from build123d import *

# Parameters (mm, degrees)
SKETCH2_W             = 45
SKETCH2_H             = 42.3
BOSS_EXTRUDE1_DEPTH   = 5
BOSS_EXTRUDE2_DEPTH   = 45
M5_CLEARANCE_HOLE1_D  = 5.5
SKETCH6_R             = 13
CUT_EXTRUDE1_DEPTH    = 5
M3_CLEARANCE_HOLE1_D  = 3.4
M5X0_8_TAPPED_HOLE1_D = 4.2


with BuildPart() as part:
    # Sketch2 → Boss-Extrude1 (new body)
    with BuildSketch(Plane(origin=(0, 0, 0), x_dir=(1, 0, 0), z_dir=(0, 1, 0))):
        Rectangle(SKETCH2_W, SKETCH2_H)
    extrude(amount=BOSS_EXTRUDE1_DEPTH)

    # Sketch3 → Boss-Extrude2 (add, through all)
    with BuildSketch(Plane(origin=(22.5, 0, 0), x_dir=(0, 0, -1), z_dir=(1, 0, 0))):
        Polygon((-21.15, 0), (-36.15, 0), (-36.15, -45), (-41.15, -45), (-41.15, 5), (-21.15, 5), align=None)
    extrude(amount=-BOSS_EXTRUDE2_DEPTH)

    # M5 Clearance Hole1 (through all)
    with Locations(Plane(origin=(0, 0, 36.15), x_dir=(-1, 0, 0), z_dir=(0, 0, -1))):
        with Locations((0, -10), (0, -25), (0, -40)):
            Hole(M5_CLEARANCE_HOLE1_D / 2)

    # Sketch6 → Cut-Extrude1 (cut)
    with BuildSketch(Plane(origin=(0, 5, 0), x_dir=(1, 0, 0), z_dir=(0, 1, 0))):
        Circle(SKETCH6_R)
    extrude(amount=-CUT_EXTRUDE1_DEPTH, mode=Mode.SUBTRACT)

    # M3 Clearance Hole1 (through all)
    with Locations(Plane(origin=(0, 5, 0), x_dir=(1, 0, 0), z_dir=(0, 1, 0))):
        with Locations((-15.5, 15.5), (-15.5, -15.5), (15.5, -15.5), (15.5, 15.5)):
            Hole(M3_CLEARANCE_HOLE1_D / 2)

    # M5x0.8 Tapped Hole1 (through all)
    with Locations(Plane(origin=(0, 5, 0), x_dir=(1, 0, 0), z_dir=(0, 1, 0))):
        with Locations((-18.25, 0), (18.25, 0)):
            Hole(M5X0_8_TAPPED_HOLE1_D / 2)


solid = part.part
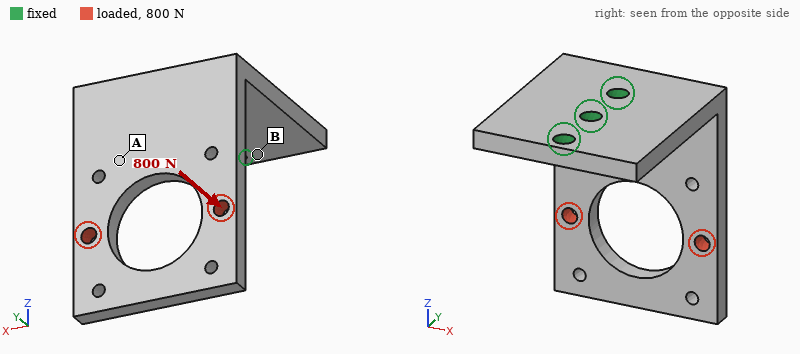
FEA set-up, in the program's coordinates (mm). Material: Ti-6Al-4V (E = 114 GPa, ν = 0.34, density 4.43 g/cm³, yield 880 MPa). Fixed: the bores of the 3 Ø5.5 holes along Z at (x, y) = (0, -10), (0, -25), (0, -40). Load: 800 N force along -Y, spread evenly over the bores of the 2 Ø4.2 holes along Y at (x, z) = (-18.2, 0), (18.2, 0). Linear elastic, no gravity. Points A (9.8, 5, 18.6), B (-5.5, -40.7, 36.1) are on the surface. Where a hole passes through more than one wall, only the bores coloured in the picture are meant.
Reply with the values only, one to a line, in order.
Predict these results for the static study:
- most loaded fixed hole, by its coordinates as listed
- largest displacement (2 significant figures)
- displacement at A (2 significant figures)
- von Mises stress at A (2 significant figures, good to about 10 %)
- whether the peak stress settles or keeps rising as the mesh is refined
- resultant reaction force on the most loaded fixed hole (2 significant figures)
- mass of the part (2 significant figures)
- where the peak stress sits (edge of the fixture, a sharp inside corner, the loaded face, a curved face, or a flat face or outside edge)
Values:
(0, -10)
0.97 mm
0.24 mm
83 MPa
keeps rising
1.1 kN
92 g
edge of the fixture
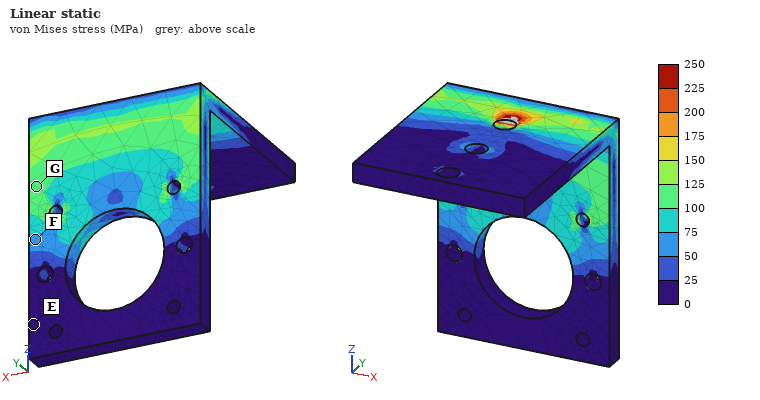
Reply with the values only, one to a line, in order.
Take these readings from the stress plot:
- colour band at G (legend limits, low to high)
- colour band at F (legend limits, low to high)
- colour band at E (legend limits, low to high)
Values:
100 to 125 MPa
50 to 75 MPa
0 to 25 MPa
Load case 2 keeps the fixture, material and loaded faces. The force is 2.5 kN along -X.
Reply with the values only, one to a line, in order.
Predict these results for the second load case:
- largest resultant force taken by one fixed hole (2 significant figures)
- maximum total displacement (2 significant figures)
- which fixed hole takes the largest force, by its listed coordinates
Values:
3.2 kN
0.95 mm
(0, -10)
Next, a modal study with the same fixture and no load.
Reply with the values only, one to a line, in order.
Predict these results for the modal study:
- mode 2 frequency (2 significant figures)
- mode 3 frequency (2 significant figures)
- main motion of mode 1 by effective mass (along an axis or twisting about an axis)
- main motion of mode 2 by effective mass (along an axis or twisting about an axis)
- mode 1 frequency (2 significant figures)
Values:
1600 Hz
2800 Hz
along Y
along X
960 Hz
